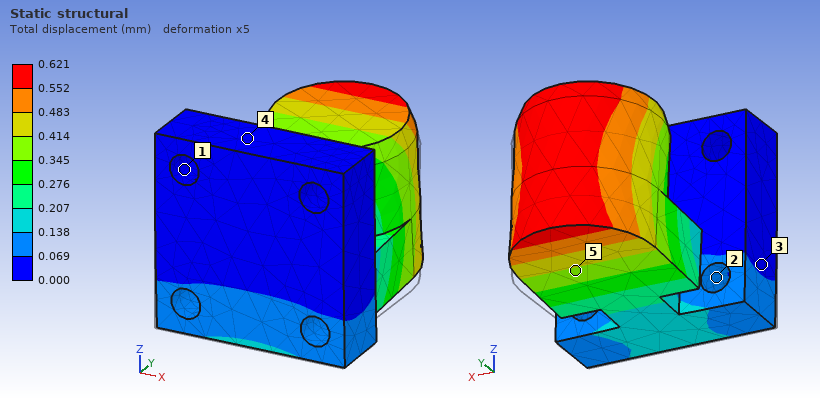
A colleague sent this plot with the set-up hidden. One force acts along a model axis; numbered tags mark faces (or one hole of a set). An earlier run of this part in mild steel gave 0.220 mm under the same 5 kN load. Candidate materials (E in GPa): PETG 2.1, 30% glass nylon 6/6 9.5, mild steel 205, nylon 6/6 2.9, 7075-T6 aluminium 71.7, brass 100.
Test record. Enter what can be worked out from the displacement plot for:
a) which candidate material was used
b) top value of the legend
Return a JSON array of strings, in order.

["7075-T6 aluminium", "0.621 mm"]
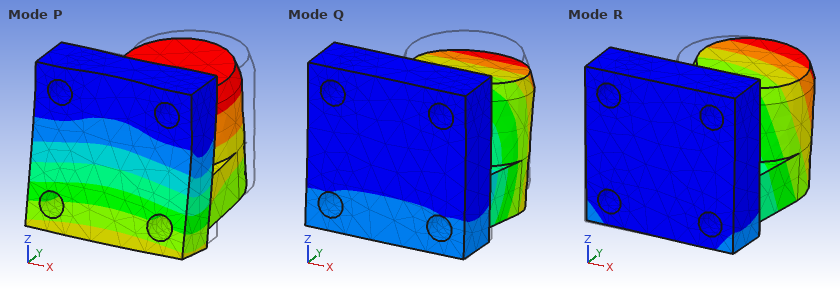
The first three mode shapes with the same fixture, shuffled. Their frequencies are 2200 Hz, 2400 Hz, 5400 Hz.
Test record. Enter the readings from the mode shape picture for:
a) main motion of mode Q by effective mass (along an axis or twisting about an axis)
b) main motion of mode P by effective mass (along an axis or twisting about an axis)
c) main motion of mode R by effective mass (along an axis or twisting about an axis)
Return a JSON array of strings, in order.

["along Z", "along Y", "along X"]
